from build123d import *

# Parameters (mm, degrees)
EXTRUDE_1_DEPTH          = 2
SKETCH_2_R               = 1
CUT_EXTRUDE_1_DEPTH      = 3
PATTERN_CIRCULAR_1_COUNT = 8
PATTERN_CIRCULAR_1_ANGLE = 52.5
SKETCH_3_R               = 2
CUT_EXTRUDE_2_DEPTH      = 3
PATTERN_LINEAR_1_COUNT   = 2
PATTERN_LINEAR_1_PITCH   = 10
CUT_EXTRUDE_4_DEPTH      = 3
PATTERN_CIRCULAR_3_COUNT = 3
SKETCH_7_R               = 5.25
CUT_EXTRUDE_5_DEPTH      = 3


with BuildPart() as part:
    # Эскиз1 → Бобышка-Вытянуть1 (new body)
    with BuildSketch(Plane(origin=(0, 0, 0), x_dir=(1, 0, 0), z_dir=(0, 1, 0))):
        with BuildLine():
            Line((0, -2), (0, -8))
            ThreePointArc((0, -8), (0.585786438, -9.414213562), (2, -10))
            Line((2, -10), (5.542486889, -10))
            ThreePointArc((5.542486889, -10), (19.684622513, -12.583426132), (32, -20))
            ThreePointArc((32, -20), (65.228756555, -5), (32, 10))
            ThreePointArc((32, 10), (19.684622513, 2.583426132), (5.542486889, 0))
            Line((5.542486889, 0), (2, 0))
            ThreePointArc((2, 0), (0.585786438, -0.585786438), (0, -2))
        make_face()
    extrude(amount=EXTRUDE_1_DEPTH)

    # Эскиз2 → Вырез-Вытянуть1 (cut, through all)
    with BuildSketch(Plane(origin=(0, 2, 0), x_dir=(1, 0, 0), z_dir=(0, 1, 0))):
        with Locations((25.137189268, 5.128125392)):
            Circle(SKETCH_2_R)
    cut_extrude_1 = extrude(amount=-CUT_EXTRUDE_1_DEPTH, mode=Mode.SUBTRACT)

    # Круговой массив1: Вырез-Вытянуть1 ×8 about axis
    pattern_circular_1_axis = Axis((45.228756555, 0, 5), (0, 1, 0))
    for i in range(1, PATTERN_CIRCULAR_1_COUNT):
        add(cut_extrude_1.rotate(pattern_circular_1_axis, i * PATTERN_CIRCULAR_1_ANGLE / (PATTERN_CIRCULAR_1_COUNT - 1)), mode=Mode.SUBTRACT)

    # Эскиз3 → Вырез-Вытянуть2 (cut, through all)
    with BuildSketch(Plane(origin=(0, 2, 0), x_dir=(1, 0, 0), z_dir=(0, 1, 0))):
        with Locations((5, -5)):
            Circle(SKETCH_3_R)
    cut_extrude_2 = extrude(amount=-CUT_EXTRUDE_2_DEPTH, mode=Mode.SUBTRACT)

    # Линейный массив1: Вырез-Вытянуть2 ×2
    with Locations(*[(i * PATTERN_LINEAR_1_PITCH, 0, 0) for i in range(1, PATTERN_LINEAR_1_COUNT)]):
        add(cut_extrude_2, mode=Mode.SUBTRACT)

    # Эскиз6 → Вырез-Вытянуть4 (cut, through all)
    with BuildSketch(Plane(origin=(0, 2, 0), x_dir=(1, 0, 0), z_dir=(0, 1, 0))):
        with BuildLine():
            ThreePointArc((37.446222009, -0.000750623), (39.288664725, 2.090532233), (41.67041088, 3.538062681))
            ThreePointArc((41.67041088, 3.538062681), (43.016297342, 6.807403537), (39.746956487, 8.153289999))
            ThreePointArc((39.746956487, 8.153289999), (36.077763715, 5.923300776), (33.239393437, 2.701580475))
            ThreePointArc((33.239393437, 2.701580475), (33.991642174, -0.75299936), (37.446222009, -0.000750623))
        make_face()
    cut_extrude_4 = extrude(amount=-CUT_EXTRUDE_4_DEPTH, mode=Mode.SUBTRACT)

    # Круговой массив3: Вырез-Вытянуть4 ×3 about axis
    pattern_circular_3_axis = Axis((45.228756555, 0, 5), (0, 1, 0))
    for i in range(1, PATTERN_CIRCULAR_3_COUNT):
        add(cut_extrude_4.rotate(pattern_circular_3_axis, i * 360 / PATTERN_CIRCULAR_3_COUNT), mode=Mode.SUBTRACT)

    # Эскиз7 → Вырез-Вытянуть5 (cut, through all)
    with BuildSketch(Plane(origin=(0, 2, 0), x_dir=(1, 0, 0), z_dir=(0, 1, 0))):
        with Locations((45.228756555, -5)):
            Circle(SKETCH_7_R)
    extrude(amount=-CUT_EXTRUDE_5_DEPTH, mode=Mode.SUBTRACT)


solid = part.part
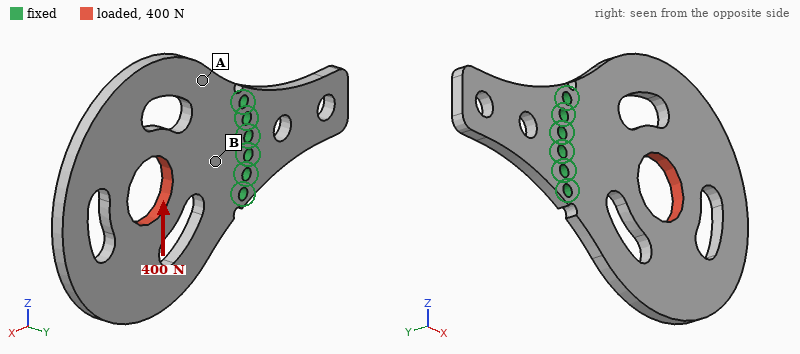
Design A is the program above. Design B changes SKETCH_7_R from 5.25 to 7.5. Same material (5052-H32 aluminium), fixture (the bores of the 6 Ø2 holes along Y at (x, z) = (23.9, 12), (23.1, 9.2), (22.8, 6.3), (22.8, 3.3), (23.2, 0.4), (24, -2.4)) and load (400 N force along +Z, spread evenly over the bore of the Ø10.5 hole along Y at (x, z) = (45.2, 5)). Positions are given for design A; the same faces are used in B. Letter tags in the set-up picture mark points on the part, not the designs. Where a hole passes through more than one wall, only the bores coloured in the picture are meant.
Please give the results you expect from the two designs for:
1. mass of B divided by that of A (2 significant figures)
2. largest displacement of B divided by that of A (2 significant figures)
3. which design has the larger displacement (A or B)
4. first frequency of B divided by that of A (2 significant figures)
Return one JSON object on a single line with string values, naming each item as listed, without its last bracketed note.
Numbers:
{"mass of B divided by that of A": "0.93", "largest displacement of B divided by that of A": "1.4", "which design has the larger displacement": "B", "first frequency of B divided by that of A": "0.96"}
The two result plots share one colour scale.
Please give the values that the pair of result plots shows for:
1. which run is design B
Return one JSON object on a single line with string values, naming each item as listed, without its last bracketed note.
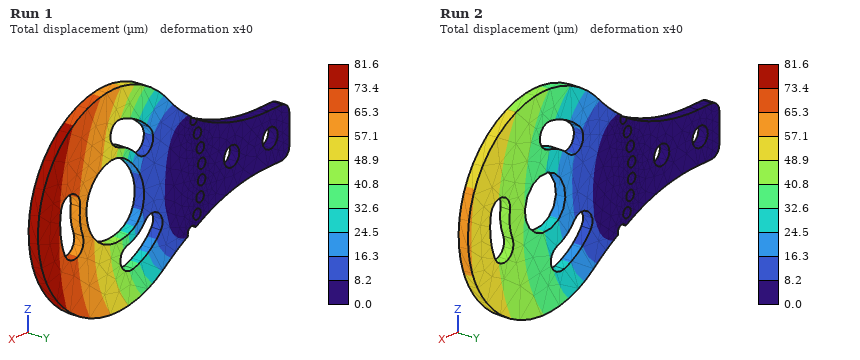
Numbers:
{"which run is design B": "Run 1"}
